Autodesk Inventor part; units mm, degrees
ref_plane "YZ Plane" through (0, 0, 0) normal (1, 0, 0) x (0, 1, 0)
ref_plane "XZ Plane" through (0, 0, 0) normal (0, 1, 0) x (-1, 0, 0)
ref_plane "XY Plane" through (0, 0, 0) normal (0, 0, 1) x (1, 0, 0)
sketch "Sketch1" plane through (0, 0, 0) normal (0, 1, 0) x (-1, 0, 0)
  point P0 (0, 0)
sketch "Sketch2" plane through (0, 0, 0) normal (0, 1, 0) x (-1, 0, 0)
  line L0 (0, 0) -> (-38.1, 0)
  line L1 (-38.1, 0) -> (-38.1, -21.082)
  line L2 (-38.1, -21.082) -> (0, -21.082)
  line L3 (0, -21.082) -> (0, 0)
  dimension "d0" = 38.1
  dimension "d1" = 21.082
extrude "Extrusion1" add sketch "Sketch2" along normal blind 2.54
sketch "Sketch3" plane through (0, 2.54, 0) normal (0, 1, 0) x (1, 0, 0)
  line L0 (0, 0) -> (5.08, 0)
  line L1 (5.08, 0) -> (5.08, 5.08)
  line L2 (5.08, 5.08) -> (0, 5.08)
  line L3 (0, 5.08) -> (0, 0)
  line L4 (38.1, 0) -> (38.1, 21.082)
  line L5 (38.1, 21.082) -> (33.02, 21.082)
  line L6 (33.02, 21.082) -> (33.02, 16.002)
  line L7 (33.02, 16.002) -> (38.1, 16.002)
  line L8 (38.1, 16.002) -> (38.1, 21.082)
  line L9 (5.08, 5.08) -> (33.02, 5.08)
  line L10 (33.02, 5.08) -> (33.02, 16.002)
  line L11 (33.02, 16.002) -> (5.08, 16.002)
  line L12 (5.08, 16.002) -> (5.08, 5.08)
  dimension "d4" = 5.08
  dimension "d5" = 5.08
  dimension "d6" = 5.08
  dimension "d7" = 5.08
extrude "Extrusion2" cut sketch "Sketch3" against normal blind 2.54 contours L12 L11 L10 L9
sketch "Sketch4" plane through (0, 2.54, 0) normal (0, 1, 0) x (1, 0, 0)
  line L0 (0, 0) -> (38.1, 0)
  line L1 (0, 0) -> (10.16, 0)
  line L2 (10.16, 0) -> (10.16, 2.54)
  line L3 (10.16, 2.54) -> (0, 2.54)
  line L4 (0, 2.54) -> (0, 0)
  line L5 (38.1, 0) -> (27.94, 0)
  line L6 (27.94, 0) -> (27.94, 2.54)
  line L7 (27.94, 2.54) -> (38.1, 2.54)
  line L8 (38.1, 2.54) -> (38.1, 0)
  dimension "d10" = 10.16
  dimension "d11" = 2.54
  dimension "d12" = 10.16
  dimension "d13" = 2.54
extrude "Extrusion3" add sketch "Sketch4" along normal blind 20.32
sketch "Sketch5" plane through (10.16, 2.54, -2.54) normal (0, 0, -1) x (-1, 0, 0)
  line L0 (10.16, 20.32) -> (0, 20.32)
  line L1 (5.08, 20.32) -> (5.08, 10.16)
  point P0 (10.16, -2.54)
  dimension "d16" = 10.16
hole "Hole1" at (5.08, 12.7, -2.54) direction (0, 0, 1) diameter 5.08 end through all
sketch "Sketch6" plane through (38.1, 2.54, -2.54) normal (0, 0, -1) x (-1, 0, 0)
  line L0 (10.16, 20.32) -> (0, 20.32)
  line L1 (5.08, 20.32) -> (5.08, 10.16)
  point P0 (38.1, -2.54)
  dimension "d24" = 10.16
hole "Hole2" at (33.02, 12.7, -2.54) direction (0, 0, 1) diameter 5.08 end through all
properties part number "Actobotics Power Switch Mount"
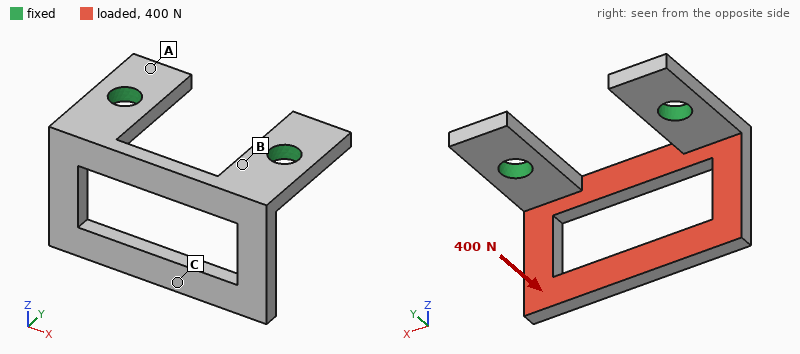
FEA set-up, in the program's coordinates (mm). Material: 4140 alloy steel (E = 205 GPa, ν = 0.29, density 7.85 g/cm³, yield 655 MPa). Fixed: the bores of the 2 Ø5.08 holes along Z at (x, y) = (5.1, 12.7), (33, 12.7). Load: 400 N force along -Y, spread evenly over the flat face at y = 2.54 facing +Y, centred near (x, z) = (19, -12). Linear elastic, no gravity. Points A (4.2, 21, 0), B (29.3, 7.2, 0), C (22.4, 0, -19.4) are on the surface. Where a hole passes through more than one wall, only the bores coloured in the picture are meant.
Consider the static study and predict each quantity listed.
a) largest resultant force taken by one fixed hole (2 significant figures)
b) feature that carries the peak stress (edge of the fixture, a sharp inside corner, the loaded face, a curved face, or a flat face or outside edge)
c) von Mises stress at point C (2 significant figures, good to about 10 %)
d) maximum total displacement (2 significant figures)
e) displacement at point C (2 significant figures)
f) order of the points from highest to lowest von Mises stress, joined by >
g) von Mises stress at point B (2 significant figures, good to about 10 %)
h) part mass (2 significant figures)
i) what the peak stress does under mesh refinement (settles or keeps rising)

200 N
a sharp inside corner
60 MPa
0.29 mm
0.26 mm
B > C > A
170 MPa
17 g
keeps rising
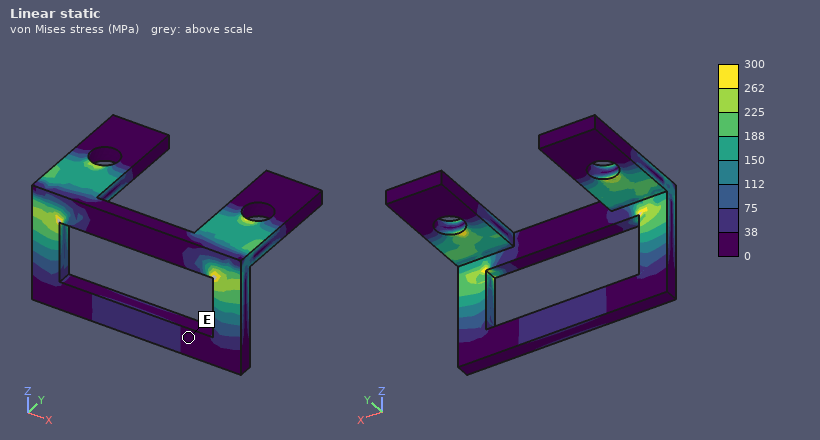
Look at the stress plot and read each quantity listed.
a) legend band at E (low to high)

0 to 38 MPa
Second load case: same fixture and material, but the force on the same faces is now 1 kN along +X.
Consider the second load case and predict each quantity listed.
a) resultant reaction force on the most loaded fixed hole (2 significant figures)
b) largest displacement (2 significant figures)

570 N
0.12 mm
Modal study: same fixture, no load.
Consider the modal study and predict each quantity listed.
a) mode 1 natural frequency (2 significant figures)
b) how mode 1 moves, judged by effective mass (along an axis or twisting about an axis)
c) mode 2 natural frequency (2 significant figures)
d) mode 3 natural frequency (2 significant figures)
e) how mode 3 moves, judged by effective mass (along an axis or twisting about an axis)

2300 Hz
along Y
4600 Hz
6700 Hz
along X
